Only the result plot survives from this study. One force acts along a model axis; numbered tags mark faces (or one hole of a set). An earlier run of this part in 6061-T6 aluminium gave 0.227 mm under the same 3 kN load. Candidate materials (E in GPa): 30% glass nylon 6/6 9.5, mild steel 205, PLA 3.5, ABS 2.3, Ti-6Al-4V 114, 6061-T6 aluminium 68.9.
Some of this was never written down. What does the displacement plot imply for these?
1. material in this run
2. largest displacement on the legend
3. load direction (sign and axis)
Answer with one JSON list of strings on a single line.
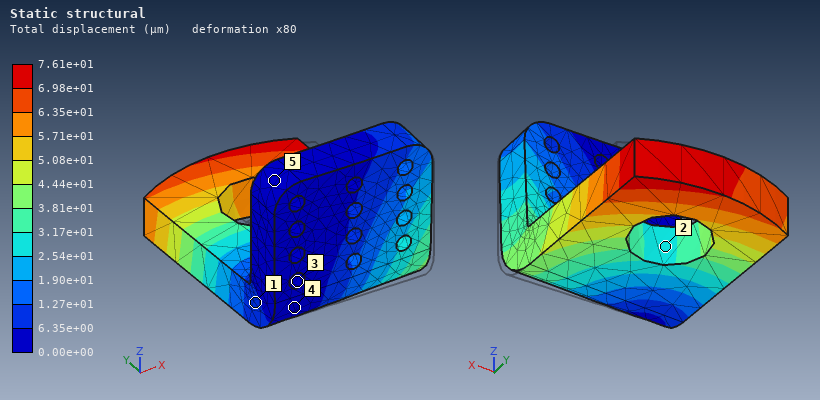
["mild steel", "7.61e+01 µm", "-X"]
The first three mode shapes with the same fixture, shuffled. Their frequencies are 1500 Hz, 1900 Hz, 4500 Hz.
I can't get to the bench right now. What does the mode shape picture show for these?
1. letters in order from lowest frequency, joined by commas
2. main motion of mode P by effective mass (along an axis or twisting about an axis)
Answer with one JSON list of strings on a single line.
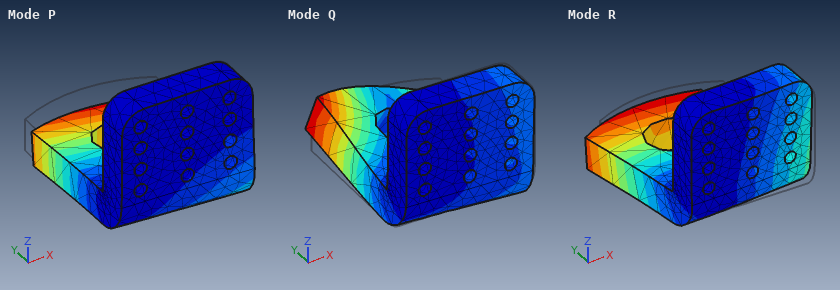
["P, R, Q", "along Z"]
